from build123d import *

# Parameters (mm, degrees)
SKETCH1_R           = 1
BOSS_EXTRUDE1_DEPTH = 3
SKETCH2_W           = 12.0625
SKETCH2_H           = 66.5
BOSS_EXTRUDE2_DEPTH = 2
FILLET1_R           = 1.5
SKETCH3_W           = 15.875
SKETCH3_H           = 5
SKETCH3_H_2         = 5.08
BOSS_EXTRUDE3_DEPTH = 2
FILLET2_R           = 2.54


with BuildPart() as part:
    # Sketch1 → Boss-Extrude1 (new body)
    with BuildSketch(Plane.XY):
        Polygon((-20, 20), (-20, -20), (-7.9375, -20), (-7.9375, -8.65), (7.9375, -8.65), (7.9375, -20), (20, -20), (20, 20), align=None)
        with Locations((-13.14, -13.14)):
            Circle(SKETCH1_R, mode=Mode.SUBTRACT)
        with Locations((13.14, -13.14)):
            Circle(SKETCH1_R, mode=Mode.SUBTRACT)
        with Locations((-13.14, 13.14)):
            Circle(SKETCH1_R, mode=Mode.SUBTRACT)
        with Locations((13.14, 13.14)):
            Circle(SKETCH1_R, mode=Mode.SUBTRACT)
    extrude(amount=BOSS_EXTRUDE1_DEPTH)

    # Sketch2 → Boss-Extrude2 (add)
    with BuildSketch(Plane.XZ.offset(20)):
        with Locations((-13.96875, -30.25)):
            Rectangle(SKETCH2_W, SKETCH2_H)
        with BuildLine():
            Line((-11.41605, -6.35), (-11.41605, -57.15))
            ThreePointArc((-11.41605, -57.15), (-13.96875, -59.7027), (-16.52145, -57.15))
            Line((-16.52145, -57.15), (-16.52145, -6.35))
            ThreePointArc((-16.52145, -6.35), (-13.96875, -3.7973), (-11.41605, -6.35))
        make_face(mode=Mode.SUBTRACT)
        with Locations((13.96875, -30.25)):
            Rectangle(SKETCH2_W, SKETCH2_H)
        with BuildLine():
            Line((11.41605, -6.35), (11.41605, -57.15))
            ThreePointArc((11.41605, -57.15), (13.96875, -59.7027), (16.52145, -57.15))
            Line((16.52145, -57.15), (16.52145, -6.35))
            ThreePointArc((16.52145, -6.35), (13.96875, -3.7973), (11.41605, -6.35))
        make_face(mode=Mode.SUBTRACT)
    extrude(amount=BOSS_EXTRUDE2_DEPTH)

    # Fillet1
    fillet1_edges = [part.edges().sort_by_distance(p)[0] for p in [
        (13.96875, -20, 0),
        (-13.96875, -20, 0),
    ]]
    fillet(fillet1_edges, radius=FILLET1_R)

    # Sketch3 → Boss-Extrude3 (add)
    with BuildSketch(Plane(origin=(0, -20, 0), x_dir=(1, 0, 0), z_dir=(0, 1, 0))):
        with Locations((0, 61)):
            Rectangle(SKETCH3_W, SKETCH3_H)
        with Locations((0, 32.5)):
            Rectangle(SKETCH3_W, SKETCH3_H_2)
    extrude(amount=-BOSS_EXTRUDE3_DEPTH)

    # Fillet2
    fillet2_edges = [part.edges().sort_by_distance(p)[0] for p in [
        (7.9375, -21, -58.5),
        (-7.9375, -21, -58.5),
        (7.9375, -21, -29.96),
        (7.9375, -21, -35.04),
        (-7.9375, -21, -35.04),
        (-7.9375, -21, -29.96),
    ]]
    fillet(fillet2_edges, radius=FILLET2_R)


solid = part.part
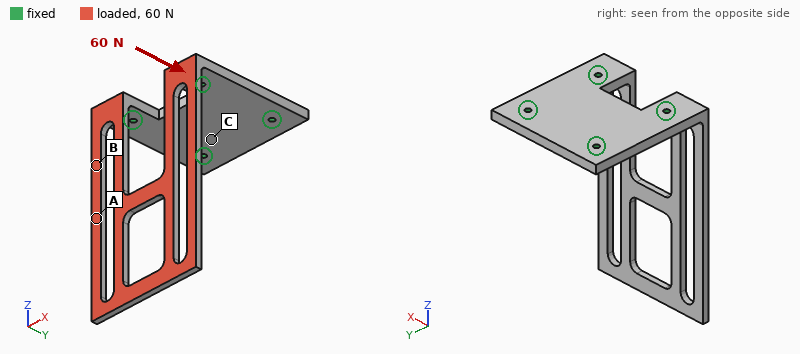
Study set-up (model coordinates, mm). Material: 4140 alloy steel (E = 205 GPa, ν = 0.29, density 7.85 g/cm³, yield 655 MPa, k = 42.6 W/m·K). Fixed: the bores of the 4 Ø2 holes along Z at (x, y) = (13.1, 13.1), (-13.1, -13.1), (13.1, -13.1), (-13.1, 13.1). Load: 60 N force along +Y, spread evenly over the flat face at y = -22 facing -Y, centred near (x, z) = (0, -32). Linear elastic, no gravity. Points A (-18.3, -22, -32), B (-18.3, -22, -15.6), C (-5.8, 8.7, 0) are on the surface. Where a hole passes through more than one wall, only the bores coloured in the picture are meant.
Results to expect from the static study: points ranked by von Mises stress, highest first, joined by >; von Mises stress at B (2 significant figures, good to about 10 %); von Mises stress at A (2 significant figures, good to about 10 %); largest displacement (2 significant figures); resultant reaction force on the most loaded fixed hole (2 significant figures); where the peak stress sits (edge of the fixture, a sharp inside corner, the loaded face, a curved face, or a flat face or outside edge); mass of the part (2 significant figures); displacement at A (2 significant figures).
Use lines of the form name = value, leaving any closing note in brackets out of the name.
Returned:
points ranked by von Mises stress, highest first, joined by > = B > A > C
von Mises stress at B = 120 MPa
von Mises stress at A = 59 MPa
largest displacement = 1.1 mm
resultant reaction force on the most loaded fixed hole = 29 N
where the peak stress sits = a curved face
mass of the part = 52 g
displacement at A = 0.37 mm
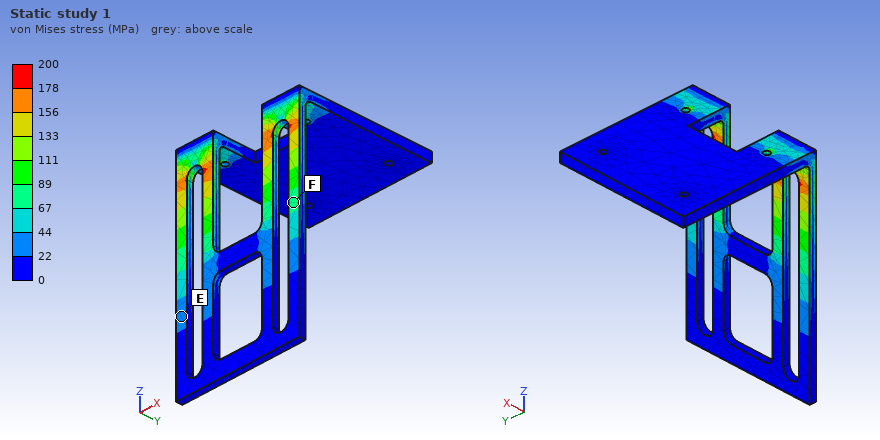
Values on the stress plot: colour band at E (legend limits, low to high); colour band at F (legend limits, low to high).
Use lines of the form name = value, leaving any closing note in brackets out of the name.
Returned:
colour band at E = 22 to 44 MPa
colour band at F = 67 to 89 MPa
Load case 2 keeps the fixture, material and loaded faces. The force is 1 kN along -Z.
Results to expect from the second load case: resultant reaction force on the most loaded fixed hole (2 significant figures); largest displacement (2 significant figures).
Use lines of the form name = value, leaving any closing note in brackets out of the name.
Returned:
resultant reaction force on the most loaded fixed hole = 530 N
largest displacement = 0.88 mm
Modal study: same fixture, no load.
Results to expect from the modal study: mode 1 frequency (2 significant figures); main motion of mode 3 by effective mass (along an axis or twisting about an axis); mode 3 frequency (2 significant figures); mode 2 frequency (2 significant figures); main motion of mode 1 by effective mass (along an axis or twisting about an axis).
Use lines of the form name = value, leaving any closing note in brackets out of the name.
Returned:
mode 1 frequency = 330 Hz
main motion of mode 3 by effective mass = along X
mode 3 frequency = 1500 Hz
mode 2 frequency = 1000 Hz
main motion of mode 1 by effective mass = along Y
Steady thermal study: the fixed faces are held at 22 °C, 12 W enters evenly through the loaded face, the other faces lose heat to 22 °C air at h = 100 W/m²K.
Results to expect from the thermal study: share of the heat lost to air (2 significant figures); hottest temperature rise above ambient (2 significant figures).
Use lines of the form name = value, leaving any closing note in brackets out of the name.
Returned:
share of the heat lost to air = 74 %
hottest temperature rise above ambient = 49 K
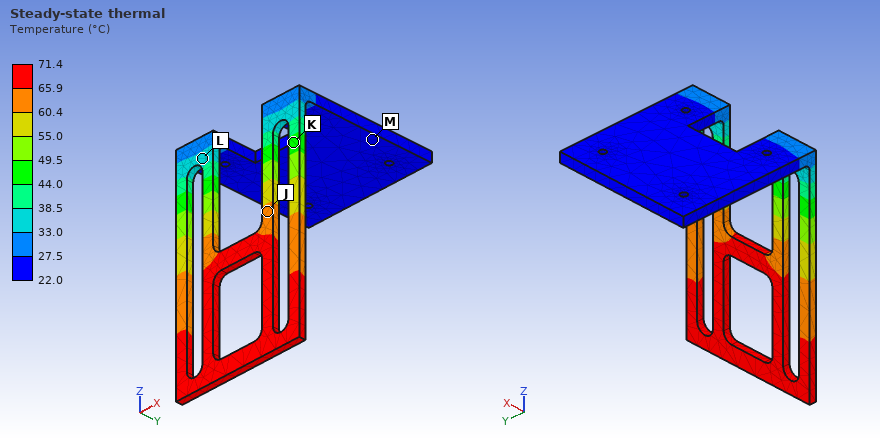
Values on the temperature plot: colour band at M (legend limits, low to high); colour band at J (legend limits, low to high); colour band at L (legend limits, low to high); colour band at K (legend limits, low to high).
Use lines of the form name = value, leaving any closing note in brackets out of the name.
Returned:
colour band at M = 22.0 to 27.5 °C
colour band at J = 60.4 to 65.9 °C
colour band at L = 33.0 to 38.5 °C
colour band at K = 44.0 to 49.5 °C
